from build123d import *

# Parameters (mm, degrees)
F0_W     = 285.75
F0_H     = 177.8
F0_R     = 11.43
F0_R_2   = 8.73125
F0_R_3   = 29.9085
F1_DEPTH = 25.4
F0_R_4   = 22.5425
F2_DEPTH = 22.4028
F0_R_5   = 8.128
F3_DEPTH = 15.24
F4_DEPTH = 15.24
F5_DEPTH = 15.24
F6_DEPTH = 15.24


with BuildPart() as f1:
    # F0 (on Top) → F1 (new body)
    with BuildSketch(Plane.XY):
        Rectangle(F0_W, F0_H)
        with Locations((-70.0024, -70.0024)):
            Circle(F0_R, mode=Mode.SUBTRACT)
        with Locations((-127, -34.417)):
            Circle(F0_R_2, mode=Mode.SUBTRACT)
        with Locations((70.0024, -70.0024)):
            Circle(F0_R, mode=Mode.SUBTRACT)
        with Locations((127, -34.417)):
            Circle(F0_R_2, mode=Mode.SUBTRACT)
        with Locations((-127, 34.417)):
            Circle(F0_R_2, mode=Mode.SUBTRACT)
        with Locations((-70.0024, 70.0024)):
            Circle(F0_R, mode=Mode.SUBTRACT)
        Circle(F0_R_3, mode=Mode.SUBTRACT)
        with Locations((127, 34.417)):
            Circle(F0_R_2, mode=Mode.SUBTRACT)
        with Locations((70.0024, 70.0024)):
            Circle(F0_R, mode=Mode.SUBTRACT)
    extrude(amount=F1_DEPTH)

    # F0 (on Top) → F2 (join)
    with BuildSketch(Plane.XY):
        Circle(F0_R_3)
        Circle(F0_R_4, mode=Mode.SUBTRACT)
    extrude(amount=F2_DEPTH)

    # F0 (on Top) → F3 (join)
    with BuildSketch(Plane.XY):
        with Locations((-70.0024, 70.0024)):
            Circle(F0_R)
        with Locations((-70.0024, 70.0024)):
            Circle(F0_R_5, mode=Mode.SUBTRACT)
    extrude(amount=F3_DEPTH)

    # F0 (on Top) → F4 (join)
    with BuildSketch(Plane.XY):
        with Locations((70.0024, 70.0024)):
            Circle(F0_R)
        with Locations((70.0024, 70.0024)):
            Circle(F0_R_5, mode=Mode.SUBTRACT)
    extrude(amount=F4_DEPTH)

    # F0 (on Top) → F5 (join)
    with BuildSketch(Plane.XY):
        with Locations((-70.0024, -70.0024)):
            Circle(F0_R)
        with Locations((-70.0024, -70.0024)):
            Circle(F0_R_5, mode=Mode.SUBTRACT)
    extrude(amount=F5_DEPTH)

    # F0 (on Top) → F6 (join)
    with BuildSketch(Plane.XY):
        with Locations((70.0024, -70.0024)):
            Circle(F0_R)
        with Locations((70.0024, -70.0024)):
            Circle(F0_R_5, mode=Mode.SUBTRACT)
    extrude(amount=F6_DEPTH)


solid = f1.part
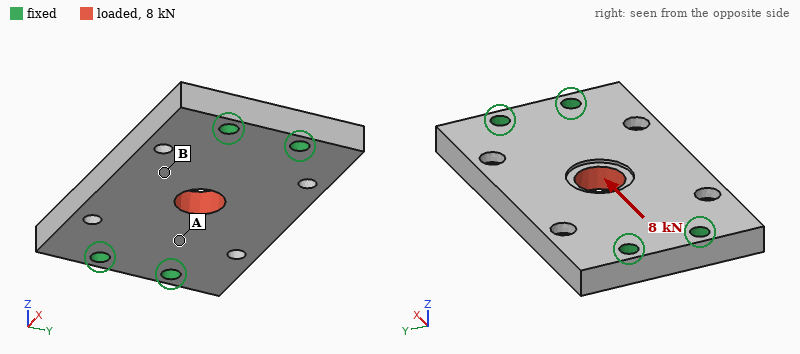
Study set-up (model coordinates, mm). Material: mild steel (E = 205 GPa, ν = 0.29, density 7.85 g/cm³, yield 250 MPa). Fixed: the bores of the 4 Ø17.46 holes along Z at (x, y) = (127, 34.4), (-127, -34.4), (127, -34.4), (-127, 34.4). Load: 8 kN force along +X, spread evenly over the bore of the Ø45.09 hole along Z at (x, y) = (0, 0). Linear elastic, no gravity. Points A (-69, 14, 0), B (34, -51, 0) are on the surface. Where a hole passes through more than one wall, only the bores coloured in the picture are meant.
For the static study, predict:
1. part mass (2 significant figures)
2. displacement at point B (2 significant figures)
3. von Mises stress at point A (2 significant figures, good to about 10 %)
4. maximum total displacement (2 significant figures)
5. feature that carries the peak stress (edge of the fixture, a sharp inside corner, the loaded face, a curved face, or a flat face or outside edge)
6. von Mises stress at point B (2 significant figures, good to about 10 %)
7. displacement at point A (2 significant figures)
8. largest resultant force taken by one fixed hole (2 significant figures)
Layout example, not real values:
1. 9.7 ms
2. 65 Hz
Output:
1. 9.4 kg
2. 0.53 µm
3. 1.7 MPa
4. 0.98 µm
5. a sharp inside corner
6. 0.70 MPa
7. 0.42 µm
8. 2.0 kN
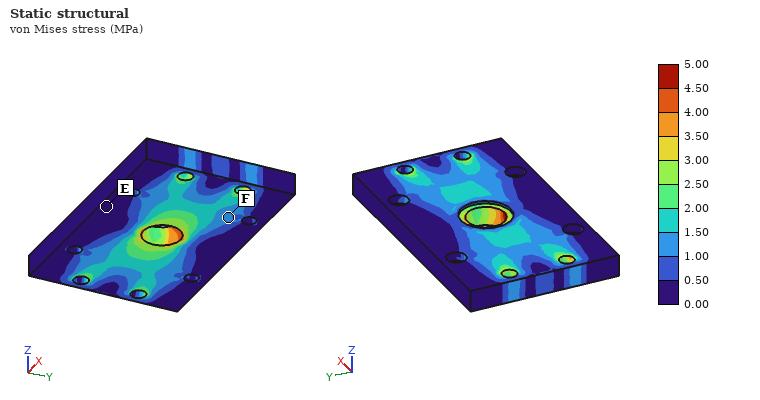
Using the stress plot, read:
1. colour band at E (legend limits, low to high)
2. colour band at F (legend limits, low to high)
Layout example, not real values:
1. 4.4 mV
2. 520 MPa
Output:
1. 0.00 to 0.50 MPa
2. 1.00 to 1.50 MPa
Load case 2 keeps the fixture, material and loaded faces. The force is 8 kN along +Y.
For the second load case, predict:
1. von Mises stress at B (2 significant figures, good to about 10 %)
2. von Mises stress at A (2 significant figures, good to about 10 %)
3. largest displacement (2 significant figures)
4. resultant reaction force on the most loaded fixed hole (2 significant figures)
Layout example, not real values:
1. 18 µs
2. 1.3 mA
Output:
1. 1.9 MPa
2. 2.6 MPa
3. 2.5 µm
4. 2.5 kN
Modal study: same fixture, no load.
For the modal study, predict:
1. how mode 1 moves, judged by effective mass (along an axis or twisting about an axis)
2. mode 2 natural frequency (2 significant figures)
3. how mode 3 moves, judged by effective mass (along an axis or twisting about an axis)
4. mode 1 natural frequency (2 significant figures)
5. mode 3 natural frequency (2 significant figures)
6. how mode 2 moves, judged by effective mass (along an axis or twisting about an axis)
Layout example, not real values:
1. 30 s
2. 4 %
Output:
1. along Z
2. 2200 Hz
3. twisting about Y
4. 1800 Hz
5. 4400 Hz
6. twisting about X
